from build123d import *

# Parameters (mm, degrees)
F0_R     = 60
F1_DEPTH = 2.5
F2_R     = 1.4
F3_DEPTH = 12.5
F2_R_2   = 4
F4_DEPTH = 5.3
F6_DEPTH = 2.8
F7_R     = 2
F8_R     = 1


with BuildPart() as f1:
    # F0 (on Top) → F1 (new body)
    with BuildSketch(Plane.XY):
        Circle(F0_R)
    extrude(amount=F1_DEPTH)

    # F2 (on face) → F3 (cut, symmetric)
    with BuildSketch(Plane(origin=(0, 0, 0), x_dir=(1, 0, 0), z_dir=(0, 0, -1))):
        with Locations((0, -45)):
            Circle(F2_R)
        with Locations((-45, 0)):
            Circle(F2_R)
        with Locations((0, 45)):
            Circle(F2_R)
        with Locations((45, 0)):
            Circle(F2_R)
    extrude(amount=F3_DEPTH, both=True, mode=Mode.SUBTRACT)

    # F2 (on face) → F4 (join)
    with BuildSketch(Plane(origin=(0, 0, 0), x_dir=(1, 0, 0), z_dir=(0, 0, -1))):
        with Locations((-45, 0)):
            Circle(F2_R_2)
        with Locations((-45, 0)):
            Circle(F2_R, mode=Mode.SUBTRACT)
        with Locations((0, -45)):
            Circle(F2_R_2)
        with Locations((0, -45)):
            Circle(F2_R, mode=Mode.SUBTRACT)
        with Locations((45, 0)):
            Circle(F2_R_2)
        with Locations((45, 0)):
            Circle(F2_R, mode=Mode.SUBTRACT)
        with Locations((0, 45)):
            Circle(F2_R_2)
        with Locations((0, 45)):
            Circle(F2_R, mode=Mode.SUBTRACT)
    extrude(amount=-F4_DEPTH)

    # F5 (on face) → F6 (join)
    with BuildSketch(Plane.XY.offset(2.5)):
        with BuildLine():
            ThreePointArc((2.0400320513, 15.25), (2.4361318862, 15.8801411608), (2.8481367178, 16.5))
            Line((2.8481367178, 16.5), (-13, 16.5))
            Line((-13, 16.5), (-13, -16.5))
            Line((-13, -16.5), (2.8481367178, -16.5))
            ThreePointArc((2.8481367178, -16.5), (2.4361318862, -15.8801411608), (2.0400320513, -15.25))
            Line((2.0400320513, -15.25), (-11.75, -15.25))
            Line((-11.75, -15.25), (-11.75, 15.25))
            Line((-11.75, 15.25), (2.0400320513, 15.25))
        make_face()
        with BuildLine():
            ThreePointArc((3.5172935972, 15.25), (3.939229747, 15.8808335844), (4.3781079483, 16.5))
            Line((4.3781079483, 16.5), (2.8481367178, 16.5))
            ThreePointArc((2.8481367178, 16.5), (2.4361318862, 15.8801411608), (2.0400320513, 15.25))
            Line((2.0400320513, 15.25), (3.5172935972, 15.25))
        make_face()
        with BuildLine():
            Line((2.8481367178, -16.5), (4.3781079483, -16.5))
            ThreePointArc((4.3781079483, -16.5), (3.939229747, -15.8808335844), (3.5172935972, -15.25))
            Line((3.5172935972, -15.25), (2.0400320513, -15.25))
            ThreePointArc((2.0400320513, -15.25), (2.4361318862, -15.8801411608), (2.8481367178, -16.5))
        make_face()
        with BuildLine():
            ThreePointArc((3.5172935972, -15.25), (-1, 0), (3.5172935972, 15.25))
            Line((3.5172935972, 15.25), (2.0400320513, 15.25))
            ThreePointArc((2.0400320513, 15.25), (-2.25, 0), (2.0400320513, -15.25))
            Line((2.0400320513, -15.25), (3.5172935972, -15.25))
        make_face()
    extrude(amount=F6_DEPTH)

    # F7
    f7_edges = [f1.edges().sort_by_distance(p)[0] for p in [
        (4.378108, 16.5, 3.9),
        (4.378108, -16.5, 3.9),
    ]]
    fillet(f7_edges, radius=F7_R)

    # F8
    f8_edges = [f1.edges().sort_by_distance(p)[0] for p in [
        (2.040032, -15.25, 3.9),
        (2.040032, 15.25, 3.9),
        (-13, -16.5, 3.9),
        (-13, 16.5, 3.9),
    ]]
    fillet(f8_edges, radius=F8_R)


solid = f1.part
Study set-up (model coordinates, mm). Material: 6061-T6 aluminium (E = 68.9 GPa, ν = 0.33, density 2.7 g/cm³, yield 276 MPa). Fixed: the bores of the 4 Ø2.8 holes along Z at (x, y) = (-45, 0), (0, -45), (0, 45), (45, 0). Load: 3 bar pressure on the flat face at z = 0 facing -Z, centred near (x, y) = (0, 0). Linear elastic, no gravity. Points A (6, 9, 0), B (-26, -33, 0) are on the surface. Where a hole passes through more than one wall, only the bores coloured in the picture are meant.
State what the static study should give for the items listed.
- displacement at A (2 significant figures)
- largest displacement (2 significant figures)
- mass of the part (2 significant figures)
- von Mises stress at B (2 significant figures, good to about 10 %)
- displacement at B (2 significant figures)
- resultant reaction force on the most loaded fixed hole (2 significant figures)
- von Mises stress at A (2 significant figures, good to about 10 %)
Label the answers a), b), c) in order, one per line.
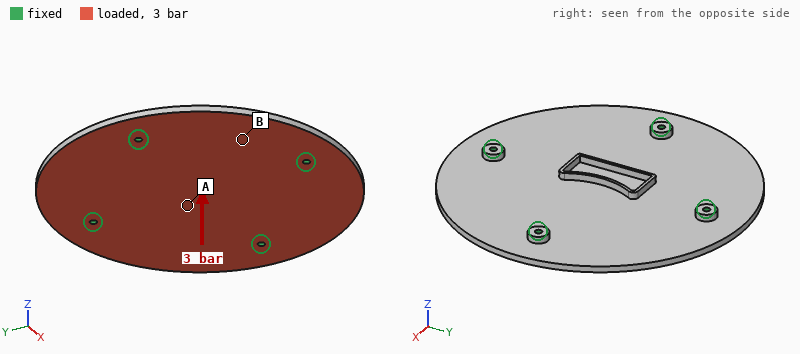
a) 0.22 mm
b) 0.32 mm
c) 78 g
d) 57 MPa
e) 0.20 mm
f) 860 N
g) 33 MPa
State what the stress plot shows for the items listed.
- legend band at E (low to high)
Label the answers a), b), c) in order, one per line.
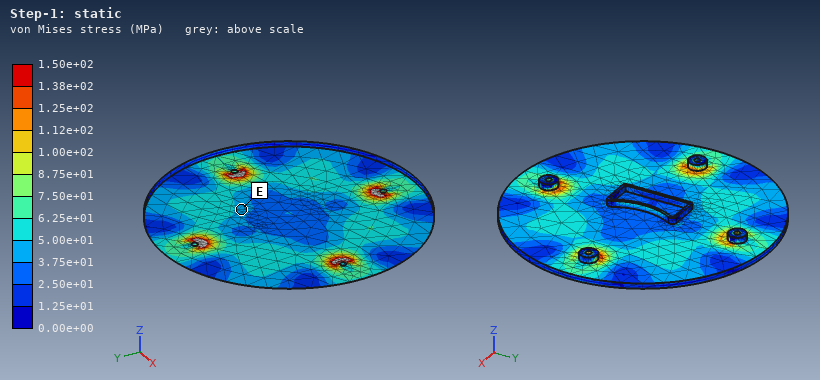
a) 3.75e+01 to 5.00e+01 MPa
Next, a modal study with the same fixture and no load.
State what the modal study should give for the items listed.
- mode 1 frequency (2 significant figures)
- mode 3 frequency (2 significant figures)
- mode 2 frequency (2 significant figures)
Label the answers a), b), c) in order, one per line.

a) 2100 Hz
b) 2200 Hz
c) 2200 Hz
